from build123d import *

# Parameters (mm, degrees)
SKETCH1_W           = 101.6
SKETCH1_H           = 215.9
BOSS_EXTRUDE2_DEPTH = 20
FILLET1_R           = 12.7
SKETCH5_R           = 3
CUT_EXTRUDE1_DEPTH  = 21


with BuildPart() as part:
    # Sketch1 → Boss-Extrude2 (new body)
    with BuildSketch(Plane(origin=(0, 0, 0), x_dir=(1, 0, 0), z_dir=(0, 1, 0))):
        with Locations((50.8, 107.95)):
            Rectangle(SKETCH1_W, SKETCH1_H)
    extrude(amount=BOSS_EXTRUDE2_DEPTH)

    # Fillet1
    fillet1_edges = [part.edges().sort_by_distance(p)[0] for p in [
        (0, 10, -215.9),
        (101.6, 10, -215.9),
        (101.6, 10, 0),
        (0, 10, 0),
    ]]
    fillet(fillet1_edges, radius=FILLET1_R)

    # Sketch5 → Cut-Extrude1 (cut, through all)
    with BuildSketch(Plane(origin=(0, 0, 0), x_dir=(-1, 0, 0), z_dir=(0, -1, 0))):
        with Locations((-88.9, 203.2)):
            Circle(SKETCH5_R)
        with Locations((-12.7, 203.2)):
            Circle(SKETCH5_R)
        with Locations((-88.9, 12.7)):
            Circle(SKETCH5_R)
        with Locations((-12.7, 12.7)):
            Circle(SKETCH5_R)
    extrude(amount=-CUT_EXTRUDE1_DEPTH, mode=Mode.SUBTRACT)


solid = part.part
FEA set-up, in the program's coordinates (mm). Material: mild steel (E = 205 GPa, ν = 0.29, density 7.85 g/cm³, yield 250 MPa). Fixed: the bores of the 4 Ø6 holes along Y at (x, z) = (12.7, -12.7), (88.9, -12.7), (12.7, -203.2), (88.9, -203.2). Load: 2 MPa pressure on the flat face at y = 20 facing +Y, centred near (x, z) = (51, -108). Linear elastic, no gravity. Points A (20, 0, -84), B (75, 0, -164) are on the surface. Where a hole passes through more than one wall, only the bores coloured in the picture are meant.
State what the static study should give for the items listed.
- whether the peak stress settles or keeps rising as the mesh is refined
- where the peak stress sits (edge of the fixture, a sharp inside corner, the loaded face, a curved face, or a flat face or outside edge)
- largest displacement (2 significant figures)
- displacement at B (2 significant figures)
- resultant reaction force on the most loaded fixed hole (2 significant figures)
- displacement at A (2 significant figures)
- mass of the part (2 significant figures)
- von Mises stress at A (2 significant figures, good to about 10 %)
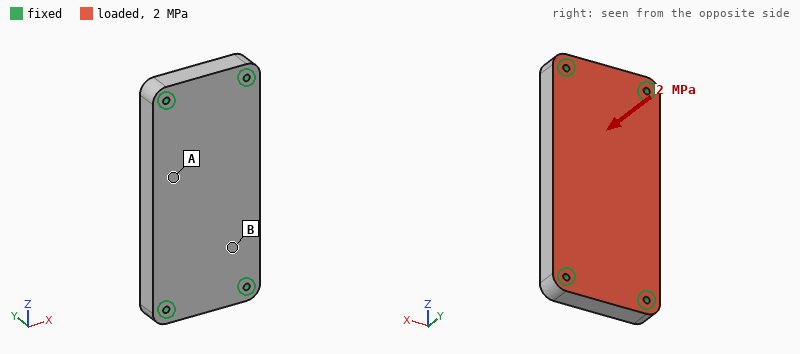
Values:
keeps rising
edge of the fixture
83 µm
44 µm
11 kN
72 µm
3.4 kg
46 MPa
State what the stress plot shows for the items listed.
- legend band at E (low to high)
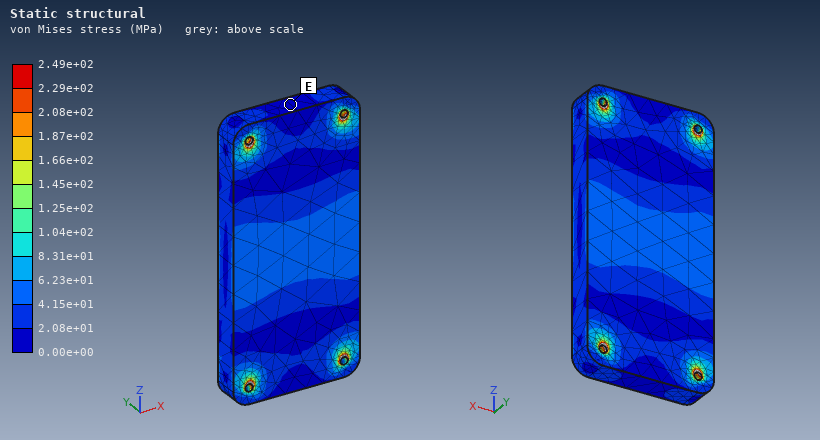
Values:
0.00e+00 to 2.08e+01 MPa
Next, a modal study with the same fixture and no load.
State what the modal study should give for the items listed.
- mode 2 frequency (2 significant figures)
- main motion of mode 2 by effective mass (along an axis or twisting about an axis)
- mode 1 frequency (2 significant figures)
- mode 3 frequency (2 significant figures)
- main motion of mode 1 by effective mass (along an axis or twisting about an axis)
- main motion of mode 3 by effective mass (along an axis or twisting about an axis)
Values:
3900 Hz
twisting about Z
2300 Hz
6000 Hz
along Y
twisting about X
